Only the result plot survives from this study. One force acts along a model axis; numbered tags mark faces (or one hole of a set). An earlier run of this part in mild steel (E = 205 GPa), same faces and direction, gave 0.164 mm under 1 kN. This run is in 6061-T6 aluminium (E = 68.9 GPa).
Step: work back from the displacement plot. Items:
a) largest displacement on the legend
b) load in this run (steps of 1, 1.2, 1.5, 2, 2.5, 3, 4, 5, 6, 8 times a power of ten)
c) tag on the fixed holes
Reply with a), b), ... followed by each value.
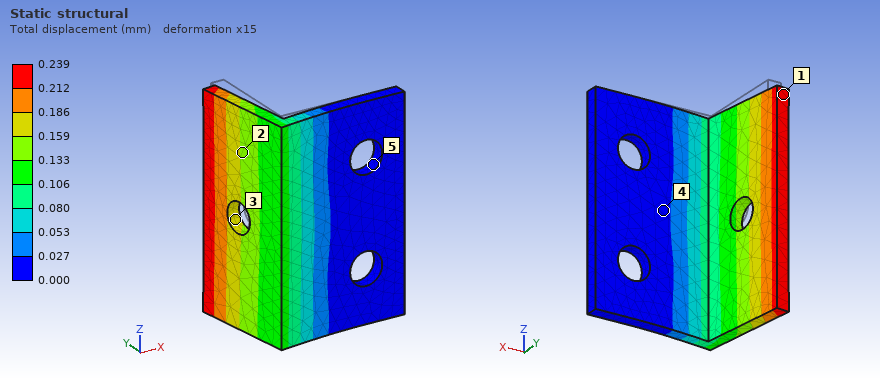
a) 0.239 mm
b) 500 N
c) 5
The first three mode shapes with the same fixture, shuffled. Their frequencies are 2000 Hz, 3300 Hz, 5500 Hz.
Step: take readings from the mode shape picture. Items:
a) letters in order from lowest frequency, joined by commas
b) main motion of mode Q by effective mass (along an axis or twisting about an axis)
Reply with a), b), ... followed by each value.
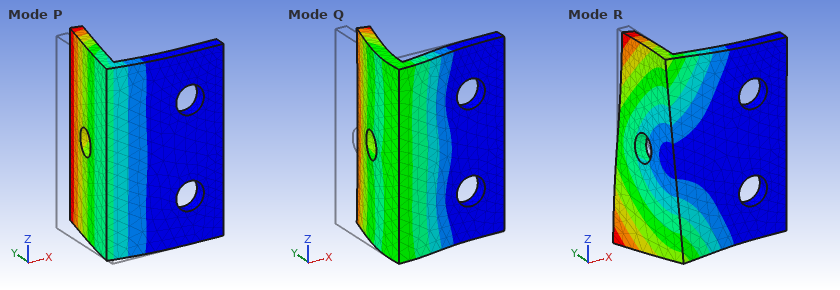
a) P, R, Q
b) along Y
